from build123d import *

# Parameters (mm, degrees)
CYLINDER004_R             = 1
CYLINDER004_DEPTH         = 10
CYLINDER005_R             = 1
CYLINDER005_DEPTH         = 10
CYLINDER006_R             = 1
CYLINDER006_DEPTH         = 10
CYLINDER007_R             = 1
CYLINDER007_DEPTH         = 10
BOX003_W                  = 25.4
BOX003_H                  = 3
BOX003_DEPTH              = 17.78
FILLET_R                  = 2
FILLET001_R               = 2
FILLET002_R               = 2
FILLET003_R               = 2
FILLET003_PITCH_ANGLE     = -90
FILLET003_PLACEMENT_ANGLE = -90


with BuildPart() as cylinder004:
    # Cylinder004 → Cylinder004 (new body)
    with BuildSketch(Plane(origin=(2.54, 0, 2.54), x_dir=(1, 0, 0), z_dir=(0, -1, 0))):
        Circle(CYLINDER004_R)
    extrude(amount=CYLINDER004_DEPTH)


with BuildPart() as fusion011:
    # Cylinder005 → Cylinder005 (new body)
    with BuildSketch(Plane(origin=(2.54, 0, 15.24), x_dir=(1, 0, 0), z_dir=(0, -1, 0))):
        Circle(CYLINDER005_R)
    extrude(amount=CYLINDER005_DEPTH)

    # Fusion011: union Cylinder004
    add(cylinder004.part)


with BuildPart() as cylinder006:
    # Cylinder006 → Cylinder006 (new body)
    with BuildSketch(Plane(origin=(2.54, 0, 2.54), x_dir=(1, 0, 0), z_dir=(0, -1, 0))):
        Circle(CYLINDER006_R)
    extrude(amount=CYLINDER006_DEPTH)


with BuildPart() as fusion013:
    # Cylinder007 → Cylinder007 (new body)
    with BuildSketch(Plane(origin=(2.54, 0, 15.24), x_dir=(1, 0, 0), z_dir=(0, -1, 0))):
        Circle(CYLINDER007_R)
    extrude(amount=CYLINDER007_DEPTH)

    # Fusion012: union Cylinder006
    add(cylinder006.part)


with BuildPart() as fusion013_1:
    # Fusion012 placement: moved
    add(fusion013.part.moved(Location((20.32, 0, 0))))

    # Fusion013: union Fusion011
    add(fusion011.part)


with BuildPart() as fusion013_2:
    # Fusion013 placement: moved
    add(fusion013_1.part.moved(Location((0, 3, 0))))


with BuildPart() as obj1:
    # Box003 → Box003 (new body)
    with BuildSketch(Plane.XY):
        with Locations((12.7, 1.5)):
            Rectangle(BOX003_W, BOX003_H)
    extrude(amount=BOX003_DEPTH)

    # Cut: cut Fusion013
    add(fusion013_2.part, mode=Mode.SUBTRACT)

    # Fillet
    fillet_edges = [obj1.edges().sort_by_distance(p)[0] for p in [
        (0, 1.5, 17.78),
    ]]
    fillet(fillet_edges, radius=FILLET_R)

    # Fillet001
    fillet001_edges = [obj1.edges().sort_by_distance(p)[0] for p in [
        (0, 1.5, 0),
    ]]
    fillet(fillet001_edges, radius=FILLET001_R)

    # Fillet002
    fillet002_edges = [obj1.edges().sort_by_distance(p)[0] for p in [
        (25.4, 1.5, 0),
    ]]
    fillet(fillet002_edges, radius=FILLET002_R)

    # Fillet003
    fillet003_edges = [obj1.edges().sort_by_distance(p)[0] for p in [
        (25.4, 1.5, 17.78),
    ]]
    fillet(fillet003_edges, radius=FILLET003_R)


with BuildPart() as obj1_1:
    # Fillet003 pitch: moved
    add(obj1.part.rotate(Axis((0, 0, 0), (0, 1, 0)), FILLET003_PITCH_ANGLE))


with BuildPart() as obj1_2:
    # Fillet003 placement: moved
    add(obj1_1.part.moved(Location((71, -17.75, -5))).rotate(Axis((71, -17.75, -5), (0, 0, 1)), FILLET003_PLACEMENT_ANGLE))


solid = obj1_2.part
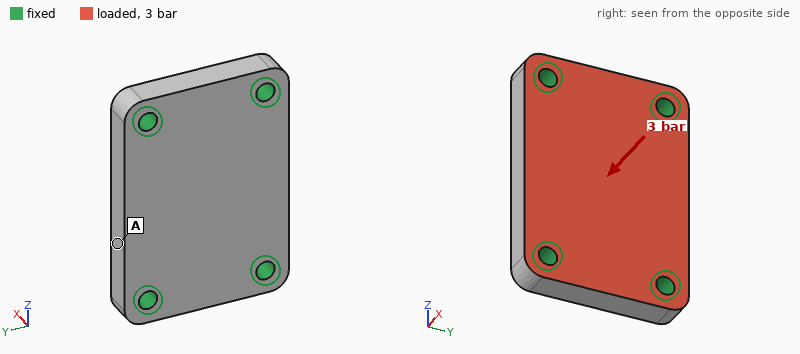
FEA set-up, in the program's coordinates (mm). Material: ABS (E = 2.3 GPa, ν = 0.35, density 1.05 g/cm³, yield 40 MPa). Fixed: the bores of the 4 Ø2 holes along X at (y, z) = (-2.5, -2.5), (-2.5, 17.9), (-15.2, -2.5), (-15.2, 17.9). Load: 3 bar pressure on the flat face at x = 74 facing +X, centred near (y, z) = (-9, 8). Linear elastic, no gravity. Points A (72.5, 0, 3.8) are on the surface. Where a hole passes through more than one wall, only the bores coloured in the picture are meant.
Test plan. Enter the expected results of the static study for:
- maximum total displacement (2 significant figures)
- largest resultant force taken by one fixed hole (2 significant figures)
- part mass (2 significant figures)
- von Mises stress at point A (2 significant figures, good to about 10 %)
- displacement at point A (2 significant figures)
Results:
38 µm
33 N
1.4 g
2.0 MPa
26 µm
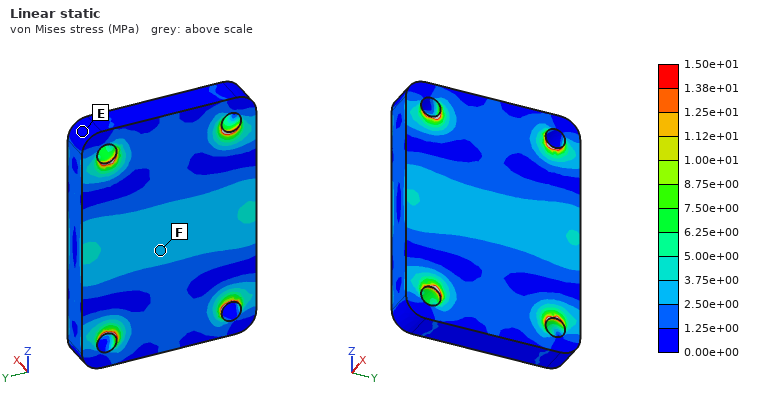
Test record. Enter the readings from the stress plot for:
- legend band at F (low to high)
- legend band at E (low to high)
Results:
2.50e+00 to 3.75e+00 MPa
0.00e+00 to 1.25e+00 MPa
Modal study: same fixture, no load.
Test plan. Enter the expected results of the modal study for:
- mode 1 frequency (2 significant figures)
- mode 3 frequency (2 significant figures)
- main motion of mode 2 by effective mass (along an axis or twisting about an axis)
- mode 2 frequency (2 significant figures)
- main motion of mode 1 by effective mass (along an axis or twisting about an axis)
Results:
9100 Hz
19 kHz
twisting about Z
12 kHz
along X
